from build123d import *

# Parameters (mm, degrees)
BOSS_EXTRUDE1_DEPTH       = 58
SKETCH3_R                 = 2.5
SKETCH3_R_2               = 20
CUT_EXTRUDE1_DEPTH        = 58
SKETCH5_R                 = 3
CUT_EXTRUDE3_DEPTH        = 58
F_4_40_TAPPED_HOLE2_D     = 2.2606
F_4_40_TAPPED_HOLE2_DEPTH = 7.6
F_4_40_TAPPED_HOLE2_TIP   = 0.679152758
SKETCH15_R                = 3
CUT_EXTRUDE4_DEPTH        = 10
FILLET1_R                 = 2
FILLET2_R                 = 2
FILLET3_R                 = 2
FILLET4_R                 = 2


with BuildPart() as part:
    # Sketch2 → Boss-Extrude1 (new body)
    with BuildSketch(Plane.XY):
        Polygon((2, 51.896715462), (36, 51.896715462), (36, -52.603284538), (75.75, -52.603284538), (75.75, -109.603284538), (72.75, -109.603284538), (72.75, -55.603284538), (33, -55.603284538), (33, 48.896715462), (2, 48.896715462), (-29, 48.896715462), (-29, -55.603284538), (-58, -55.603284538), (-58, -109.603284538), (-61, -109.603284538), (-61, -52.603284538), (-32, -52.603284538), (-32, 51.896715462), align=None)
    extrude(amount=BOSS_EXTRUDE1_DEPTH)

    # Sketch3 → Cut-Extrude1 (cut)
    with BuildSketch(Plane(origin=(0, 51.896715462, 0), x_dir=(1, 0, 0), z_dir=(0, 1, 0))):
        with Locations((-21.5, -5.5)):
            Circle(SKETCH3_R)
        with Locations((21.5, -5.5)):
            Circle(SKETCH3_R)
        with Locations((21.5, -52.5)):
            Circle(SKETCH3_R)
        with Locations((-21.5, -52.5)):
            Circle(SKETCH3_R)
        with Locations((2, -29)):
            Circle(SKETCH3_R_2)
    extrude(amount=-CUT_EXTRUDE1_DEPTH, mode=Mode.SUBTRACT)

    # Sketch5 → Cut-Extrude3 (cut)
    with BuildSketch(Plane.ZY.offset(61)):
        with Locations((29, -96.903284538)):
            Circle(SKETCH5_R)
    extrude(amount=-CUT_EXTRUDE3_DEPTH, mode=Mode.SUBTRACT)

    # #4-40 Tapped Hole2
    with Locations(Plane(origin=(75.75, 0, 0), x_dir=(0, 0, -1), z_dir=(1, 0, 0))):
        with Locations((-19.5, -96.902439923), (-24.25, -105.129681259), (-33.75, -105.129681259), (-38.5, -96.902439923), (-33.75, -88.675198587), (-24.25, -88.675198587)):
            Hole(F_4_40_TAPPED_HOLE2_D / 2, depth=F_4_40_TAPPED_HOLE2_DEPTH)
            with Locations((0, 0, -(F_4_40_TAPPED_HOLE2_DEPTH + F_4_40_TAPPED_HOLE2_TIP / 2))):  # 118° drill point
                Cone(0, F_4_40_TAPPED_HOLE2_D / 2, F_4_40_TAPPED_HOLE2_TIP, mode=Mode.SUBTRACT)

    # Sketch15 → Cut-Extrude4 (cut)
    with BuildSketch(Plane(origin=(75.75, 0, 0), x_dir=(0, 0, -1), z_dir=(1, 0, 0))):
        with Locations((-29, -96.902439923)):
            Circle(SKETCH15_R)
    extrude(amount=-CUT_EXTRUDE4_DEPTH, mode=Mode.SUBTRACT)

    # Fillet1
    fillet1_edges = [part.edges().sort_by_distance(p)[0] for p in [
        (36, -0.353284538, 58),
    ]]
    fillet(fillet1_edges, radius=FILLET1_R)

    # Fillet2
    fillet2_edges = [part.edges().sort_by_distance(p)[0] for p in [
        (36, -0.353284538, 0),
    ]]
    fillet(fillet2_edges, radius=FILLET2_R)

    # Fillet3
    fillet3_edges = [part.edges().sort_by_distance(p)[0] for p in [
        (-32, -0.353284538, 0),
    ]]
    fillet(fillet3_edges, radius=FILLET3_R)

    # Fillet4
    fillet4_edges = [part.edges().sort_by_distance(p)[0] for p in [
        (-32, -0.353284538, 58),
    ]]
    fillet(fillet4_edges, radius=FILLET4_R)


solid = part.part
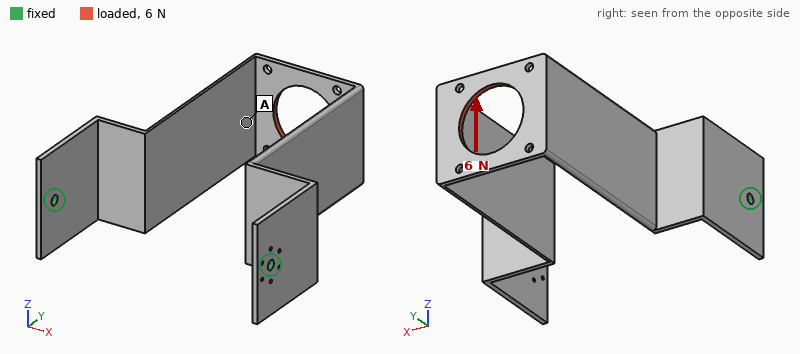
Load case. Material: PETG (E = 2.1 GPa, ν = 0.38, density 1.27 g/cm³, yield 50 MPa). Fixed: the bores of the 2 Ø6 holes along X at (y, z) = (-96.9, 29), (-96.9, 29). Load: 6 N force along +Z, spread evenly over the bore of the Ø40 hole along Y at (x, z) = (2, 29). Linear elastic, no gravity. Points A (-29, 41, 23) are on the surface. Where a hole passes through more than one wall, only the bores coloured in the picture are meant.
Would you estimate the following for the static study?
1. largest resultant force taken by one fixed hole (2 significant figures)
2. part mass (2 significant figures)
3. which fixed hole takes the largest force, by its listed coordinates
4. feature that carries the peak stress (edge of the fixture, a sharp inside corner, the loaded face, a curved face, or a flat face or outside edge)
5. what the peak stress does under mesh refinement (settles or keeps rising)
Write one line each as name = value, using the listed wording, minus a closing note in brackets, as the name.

largest resultant force taken by one fixed hole = 3.4 N
part mass = 94 g
which fixed hole takes the largest force, by its listed coordinates = (-96.9, 29)
feature that carries the peak stress = edge of the fixture
what the peak stress does under mesh refinement = keeps rising
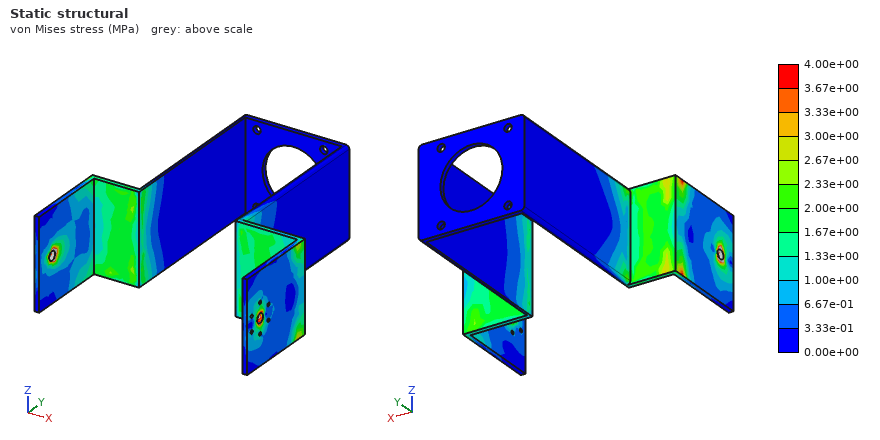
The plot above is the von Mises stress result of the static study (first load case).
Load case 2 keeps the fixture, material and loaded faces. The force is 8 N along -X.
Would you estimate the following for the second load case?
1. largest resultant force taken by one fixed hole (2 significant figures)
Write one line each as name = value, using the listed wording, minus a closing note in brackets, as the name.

largest resultant force taken by one fixed hole = 8.2 N
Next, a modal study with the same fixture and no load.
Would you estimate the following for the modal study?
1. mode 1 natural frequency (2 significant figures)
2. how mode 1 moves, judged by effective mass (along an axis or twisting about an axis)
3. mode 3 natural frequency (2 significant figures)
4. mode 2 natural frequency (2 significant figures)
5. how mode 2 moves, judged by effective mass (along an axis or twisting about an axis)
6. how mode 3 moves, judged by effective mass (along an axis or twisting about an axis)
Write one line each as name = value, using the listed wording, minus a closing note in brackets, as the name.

mode 1 natural frequency = 50 Hz
how mode 1 moves, judged by effective mass = along X
mode 3 natural frequency = 86 Hz
mode 2 natural frequency = 53 Hz
how mode 2 moves, judged by effective mass = along Z
how mode 3 moves, judged by effective mass = along Y
